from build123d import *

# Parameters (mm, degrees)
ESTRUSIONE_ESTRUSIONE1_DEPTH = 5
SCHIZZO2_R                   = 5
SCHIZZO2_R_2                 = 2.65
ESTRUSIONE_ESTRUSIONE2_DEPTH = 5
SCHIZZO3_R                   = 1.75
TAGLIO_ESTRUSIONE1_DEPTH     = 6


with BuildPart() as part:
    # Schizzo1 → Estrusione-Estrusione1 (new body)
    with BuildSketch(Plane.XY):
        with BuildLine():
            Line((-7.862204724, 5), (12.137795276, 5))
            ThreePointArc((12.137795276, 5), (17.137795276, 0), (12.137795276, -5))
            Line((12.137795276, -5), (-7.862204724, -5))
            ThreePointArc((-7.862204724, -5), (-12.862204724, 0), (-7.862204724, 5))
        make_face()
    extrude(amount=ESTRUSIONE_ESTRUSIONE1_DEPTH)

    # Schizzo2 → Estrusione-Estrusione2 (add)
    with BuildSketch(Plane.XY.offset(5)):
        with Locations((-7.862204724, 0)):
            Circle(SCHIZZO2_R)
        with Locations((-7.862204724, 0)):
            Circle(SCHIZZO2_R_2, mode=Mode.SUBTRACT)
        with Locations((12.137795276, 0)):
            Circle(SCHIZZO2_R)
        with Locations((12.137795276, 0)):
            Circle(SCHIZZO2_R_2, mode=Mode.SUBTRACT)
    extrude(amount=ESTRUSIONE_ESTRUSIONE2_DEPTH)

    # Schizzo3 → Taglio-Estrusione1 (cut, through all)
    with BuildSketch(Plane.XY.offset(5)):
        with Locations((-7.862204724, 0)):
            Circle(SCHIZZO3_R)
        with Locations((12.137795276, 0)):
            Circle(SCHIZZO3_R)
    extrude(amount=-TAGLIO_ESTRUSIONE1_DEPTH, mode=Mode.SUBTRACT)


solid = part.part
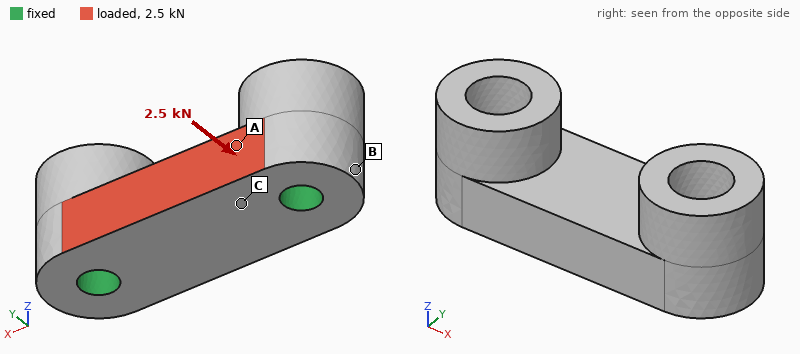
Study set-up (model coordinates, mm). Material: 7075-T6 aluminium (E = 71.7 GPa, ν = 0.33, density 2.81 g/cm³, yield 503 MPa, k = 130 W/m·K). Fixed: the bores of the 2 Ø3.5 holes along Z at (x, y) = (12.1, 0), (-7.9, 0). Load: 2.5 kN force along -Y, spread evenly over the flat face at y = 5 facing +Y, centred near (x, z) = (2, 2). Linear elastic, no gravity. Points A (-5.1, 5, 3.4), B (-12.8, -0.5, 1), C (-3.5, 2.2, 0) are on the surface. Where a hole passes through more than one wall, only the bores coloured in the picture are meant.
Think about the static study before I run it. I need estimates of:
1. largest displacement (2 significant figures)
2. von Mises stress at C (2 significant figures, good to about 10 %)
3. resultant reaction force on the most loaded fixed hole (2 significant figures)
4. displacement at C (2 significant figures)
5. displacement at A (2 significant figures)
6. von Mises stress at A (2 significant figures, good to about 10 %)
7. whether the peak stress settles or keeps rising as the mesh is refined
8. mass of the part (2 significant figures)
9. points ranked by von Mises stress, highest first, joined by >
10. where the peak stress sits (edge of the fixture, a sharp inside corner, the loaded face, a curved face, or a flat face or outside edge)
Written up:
8.3 µm
36 MPa
1.3 kN
4.6 µm
4.2 µm
23 MPa
keeps rising
5.2 g
C > A > B
edge of the fixture
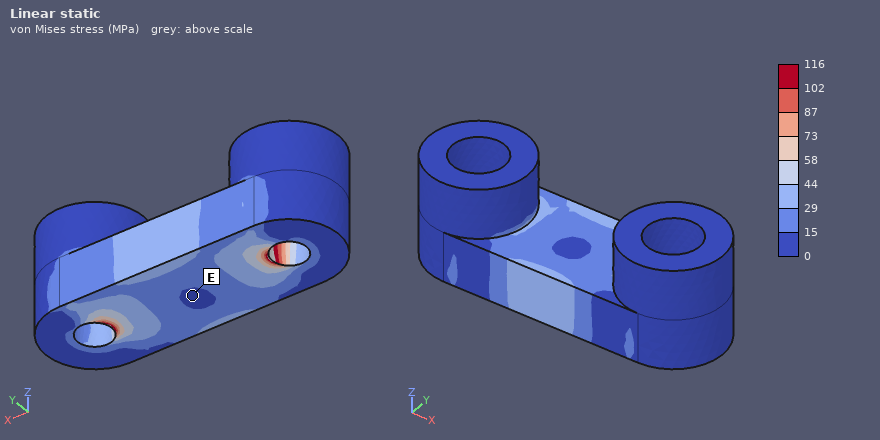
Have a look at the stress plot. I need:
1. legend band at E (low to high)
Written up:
0 to 15 MPa
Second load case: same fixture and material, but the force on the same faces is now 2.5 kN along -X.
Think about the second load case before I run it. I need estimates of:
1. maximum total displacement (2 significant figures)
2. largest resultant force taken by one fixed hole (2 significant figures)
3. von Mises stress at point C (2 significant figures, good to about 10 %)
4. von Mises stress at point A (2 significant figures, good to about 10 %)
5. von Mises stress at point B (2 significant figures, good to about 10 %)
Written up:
4.7 µm
1.4 kN
38 MPa
46 MPa
8.7 MPa
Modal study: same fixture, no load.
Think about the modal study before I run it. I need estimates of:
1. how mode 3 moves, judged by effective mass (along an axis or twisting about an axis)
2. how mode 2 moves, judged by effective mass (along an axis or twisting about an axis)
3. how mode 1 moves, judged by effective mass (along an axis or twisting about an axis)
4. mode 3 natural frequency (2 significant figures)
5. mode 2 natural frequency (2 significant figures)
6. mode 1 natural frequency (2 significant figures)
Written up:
along Y
along Y
along Z
58 kHz
53 kHz
47 kHz
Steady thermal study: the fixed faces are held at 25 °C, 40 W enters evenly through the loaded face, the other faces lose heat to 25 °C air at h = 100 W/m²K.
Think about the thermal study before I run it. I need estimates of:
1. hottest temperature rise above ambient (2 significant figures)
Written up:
23 K
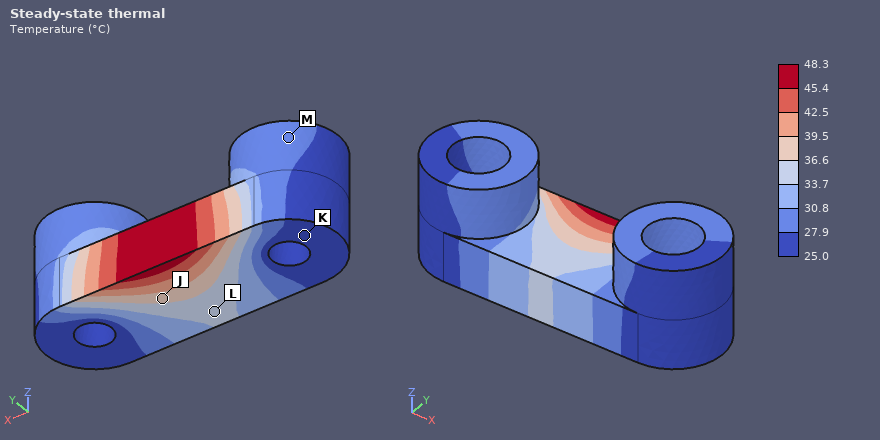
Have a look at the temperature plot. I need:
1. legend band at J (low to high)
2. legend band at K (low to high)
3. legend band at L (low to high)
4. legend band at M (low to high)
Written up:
36.6 to 39.5 °C
25.0 to 27.9 °C
33.7 to 36.6 °C
27.9 to 30.8 °C
